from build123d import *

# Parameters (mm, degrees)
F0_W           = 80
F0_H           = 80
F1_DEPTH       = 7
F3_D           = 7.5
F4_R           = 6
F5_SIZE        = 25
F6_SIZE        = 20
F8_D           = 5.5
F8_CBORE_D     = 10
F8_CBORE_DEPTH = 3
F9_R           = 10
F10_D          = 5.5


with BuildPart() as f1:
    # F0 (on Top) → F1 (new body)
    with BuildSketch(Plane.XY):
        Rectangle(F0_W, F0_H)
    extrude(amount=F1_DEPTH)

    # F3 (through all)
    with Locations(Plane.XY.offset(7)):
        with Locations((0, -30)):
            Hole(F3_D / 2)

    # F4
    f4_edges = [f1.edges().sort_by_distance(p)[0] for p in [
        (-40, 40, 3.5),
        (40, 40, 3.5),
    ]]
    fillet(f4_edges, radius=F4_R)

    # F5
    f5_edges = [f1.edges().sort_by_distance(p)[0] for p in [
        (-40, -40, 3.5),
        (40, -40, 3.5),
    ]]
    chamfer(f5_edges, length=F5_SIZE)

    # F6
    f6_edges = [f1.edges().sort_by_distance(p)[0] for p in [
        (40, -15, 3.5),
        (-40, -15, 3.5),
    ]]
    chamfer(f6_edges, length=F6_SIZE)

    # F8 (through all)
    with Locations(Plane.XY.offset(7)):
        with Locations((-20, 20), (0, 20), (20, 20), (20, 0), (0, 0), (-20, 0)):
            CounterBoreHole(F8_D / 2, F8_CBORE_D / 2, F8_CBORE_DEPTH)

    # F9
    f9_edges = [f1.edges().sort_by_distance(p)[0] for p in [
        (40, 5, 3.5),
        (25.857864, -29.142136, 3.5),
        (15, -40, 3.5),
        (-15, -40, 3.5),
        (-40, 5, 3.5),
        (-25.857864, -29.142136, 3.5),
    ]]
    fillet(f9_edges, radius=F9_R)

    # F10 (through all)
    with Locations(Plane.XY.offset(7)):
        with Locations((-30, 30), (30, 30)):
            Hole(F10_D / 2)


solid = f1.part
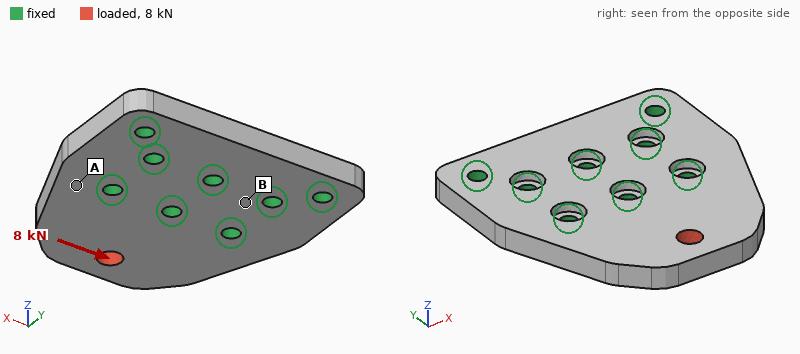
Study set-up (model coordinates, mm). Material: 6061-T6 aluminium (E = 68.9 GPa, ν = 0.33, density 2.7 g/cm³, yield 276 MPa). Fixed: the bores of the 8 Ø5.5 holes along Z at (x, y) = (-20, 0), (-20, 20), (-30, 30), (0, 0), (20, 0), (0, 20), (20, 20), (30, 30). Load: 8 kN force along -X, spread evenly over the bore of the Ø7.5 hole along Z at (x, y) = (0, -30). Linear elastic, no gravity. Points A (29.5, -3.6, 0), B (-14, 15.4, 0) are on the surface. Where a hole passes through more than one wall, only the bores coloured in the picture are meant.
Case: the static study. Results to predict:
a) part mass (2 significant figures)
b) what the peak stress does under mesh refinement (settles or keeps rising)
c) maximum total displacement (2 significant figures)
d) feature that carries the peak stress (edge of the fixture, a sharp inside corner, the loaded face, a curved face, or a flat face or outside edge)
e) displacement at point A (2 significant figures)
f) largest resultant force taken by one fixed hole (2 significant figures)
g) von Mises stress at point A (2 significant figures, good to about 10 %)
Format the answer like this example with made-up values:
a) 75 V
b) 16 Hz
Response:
a) 96 g
b) keeps rising
c) 44 µm
d) edge of the fixture
e) 8.3 µm
f) 4.1 kN
g) 26 MPa
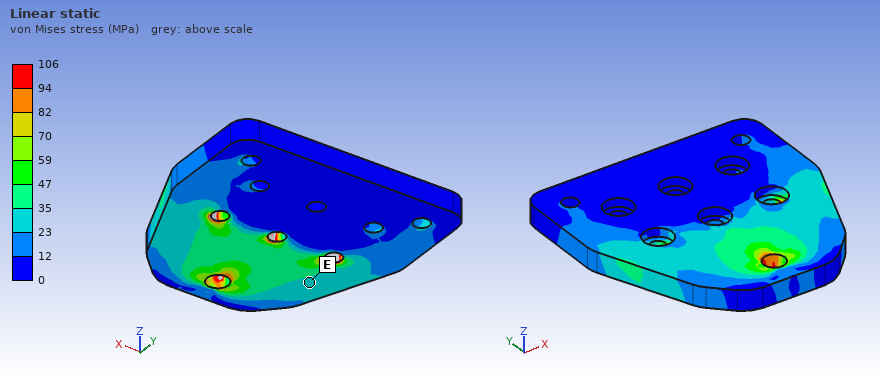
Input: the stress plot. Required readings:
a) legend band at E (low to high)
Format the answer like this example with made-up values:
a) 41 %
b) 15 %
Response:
a) 23 to 35 MPa
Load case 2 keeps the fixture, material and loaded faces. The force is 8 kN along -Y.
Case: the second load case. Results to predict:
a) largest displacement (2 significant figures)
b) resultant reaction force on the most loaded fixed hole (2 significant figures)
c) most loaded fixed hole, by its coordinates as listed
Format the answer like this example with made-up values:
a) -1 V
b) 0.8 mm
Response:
a) 35 µm
b) 2.5 kN
c) (0, 0)
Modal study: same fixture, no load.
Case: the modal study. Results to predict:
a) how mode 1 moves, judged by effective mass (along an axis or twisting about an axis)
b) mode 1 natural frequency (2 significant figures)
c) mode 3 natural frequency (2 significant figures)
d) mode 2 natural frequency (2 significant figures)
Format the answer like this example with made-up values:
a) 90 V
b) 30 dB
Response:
a) along Z
b) 3800 Hz
c) 14 kHz
d) 7800 Hz
